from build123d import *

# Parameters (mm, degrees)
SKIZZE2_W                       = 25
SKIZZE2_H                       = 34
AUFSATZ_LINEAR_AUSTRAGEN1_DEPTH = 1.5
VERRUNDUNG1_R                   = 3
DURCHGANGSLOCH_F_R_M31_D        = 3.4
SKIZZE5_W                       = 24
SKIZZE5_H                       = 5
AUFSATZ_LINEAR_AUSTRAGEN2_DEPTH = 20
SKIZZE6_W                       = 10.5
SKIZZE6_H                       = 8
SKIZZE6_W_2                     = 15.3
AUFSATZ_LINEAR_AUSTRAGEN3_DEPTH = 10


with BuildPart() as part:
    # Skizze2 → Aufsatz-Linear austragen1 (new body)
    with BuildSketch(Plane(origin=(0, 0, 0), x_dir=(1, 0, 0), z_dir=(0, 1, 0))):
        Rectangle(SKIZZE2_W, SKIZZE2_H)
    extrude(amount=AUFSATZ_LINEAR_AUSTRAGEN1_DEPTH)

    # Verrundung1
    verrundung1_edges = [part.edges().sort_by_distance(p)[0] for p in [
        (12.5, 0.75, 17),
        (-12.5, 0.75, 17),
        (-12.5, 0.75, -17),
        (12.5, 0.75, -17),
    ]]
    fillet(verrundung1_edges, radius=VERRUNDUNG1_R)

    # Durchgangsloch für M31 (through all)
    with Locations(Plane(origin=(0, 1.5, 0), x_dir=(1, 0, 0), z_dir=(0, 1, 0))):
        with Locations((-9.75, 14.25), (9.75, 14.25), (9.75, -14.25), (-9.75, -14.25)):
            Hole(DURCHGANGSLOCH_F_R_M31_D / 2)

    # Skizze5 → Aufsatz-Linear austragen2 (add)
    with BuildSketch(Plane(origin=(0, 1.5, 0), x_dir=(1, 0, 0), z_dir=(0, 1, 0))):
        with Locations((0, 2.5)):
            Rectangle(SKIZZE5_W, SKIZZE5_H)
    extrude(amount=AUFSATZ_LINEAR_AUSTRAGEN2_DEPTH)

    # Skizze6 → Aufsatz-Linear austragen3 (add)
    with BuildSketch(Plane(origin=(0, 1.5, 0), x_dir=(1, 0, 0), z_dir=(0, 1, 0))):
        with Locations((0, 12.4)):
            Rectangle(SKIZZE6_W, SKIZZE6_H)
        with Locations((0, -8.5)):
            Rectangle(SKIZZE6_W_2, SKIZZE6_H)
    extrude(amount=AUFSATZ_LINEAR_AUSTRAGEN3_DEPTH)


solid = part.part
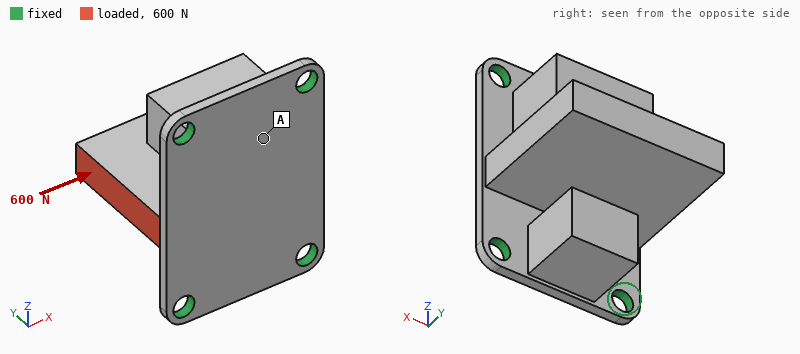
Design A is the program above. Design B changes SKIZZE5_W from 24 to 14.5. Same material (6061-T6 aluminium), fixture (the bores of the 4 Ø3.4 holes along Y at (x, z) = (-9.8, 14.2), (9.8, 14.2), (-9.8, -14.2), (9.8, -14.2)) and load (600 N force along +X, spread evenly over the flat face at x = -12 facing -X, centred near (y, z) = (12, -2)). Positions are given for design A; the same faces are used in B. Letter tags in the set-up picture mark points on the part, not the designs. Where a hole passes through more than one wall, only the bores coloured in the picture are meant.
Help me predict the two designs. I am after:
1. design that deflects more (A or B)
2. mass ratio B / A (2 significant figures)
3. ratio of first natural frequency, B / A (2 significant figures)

B
0.83
1.1
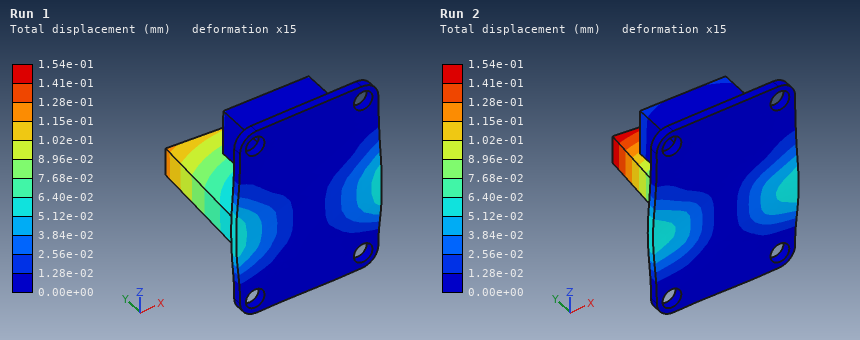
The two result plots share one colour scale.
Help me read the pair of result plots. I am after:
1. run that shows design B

Run 2
